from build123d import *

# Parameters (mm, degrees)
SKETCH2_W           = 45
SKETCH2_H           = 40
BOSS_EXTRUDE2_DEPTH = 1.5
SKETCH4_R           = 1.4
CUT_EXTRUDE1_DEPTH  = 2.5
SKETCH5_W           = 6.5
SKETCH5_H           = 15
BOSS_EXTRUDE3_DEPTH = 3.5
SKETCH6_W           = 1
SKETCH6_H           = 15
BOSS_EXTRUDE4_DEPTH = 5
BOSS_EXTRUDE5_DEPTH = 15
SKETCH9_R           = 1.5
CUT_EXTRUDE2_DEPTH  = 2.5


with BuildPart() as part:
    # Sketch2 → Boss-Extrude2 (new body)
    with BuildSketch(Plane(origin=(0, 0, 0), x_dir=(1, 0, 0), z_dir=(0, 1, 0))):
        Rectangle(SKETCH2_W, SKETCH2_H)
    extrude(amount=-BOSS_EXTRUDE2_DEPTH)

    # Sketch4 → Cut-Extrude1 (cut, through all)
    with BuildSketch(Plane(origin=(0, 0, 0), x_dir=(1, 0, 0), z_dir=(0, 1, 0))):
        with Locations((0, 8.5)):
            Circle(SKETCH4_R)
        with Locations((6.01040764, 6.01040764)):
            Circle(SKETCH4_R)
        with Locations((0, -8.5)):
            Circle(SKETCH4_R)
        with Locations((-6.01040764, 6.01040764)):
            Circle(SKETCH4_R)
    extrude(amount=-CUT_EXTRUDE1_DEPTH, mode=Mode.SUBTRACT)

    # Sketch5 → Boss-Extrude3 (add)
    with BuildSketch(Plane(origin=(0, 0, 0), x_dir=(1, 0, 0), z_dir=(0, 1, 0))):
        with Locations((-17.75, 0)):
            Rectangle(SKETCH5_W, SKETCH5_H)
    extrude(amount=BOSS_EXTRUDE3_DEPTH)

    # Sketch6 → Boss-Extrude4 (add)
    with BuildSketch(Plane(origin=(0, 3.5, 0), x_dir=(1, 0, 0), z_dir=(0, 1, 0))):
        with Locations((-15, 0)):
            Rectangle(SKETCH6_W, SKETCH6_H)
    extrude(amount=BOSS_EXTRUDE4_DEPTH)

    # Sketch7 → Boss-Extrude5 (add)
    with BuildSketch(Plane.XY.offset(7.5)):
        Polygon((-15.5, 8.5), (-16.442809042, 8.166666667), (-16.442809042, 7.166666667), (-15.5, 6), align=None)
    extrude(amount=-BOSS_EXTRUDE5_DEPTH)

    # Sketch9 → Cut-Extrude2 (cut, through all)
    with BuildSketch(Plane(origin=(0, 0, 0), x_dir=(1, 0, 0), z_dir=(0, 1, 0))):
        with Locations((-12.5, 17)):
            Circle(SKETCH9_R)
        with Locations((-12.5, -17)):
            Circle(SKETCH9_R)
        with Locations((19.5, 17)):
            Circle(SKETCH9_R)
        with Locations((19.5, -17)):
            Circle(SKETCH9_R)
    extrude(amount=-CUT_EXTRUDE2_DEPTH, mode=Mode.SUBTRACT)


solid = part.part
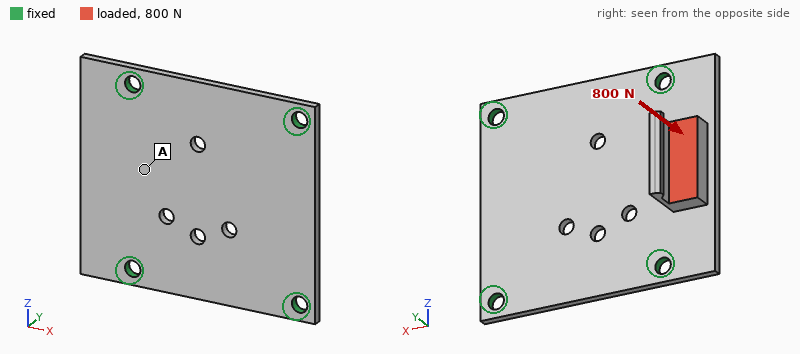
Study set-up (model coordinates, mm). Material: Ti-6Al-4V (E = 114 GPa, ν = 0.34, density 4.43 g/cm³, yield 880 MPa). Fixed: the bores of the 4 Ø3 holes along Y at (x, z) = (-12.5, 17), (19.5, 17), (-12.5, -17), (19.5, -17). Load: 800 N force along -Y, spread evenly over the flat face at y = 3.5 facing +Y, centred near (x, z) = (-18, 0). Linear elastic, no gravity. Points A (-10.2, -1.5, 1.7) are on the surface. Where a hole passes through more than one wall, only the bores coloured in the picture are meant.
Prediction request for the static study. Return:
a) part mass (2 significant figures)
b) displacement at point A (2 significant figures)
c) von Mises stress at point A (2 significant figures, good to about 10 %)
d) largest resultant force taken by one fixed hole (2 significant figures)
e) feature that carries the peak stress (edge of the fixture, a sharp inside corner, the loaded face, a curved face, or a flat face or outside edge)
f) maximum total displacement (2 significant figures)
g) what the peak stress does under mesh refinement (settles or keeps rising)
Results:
14 g
0.055 mm
93 MPa
470 N
edge of the fixture
0.26 mm
keeps rising
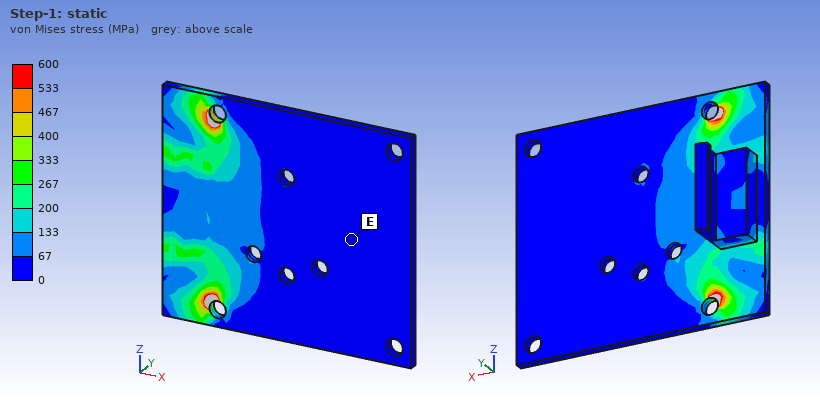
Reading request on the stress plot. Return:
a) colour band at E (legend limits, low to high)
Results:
0 to 67 MPa
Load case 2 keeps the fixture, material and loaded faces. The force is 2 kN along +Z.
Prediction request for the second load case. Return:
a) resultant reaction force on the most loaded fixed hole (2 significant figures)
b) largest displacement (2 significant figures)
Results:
1.0 kN
90 µm
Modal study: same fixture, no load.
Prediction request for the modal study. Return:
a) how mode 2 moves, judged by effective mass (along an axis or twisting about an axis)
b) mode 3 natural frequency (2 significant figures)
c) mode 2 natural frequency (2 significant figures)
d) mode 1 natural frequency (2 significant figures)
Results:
along Y
8700 Hz
5800 Hz
5200 Hz
